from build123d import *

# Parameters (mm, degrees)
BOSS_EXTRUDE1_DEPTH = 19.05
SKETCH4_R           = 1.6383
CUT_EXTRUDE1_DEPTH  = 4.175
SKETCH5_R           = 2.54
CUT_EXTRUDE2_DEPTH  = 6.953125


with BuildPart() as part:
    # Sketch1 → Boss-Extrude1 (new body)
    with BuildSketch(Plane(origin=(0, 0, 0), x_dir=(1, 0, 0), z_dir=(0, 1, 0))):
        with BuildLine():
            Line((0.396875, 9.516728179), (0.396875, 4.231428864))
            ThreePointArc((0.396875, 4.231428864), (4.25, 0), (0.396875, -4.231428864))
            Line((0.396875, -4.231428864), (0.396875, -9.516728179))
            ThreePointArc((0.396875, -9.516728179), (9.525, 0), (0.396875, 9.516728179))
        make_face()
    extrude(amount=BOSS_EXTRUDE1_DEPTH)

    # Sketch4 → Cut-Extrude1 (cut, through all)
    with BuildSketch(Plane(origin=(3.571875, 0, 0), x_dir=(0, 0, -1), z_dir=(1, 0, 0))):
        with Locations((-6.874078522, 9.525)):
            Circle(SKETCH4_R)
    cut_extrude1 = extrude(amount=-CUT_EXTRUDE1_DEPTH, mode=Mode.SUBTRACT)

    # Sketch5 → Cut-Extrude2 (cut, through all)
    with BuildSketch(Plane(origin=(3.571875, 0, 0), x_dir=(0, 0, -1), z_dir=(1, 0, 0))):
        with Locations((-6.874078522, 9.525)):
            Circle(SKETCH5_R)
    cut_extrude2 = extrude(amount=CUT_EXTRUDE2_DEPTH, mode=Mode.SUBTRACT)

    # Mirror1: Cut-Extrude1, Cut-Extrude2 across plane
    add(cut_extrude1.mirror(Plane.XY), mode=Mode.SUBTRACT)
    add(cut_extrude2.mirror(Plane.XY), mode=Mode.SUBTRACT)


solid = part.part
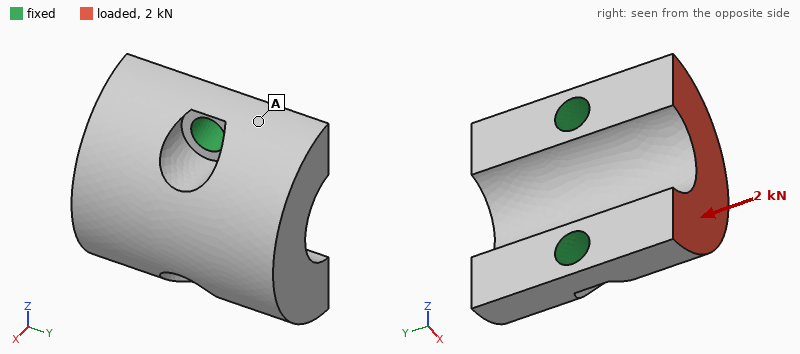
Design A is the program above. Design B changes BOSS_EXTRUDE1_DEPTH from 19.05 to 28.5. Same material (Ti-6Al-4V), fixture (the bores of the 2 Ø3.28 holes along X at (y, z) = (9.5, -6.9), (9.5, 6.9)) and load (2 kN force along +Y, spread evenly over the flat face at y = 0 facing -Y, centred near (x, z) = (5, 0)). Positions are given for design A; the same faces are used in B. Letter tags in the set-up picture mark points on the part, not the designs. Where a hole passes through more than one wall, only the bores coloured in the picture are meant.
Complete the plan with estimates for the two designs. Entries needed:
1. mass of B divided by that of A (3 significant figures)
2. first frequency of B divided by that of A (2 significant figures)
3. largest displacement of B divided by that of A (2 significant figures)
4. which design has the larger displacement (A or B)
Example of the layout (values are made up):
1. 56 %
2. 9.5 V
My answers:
1. 1.54
2. 0.47
3. 1.5
4. B
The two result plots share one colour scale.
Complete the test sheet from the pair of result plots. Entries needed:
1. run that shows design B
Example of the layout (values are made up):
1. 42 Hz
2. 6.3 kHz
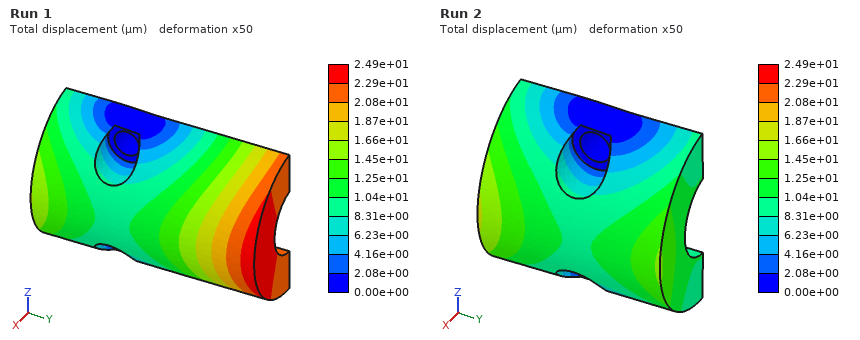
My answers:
1. Run 1
